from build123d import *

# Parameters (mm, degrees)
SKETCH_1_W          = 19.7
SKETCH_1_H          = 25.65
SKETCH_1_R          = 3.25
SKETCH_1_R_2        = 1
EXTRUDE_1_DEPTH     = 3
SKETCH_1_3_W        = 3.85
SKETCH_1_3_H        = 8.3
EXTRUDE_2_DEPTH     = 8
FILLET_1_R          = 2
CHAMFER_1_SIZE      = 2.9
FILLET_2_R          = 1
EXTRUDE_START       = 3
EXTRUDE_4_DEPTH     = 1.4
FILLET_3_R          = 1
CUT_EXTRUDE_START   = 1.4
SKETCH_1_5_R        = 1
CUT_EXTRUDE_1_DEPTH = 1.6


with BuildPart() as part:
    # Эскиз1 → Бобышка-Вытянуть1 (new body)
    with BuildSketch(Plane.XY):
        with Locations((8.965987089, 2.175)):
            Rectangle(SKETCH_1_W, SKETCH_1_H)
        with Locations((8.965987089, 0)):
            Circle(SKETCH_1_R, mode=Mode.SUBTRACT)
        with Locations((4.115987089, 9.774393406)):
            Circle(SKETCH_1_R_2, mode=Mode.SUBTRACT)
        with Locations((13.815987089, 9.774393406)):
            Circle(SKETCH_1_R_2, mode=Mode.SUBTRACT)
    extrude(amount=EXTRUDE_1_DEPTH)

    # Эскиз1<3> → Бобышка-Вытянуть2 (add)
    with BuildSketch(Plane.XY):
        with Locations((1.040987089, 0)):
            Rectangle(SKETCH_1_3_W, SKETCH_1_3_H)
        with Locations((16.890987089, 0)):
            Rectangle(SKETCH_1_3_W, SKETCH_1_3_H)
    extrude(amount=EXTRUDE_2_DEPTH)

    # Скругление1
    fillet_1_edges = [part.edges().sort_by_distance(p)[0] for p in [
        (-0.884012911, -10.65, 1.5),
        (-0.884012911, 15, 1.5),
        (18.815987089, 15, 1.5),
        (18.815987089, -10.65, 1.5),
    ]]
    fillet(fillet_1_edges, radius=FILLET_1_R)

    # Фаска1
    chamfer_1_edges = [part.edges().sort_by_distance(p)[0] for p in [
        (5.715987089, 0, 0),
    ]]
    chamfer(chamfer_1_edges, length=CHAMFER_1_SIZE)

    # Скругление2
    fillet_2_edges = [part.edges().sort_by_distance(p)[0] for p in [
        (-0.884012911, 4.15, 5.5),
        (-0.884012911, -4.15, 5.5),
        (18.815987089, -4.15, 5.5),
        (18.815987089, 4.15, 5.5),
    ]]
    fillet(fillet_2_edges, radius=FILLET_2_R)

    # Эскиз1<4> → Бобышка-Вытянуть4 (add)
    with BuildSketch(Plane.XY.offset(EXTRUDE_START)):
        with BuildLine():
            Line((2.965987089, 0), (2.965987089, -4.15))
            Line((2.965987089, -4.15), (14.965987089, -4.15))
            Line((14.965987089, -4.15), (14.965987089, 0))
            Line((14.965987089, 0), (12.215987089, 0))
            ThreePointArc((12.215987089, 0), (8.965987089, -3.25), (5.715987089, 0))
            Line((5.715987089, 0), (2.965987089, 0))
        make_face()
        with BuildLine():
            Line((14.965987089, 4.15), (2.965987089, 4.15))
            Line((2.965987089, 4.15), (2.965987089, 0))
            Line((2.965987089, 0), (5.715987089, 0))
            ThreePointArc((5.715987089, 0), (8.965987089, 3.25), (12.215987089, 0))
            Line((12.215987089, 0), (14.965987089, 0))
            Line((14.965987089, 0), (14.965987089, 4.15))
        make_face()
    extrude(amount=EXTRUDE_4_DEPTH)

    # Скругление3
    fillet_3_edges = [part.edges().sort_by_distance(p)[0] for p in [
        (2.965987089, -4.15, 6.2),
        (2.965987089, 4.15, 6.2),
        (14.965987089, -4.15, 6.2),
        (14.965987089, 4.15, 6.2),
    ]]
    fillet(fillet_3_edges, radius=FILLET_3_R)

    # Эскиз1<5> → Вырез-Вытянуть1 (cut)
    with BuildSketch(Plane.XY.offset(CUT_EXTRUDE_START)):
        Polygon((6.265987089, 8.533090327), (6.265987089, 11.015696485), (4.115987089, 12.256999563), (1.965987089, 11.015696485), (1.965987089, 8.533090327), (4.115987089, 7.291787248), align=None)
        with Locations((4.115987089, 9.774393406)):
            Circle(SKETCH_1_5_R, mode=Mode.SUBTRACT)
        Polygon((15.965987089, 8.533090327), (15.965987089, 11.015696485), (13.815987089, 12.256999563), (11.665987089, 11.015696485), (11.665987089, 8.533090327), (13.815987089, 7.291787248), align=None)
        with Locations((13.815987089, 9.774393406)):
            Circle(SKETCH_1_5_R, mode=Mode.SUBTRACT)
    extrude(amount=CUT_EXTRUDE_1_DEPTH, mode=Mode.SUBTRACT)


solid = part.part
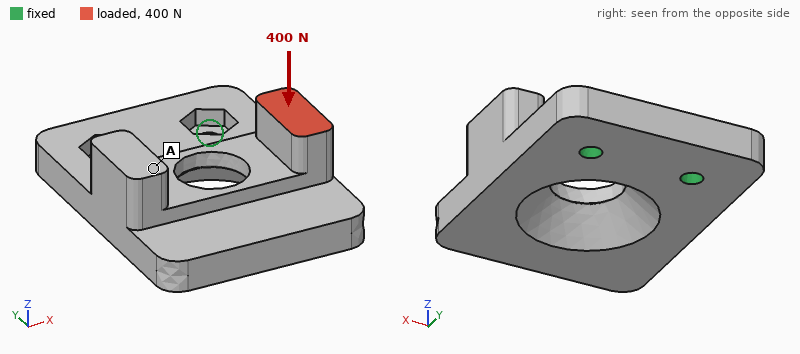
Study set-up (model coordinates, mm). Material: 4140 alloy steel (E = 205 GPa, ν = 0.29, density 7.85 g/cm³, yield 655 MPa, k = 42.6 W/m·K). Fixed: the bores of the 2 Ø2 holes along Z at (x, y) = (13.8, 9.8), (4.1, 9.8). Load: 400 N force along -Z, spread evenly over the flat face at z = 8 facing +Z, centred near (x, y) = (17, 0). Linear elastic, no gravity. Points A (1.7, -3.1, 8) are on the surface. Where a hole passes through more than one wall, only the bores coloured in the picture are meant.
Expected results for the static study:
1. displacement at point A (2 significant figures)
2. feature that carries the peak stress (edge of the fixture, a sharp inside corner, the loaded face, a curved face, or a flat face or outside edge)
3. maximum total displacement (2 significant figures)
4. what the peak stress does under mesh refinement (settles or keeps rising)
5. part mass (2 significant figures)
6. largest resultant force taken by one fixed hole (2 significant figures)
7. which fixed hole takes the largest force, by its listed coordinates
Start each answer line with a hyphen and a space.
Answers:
- 0.054 mm
- edge of the fixture
- 0.12 mm
- keeps rising
- 13 g
- 480 N
- (13.8, 9.8)
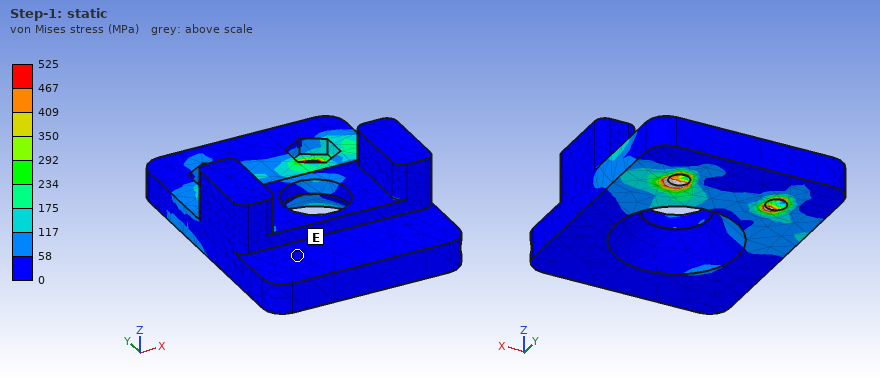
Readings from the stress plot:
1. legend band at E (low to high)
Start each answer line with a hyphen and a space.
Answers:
- 0 to 58 MPa
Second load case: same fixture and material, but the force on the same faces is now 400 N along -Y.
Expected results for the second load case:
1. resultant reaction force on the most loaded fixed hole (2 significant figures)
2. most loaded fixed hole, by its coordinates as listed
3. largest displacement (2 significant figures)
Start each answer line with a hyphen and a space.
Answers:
- 480 N
- (13.8, 9.8)
- 0.10 mm
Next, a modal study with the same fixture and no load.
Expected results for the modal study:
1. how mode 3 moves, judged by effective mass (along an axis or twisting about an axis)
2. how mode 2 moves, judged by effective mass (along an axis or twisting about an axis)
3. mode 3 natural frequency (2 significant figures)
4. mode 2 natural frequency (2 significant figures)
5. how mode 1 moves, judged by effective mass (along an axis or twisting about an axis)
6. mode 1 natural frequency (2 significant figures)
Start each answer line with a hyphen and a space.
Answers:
- along X
- twisting about Y
- 14 kHz
- 9300 Hz
- along Z
- 3600 Hz
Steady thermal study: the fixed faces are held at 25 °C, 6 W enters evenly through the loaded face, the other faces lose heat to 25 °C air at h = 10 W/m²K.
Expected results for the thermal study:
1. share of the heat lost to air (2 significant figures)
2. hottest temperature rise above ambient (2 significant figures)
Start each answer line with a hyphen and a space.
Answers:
- 5.5 %
- 65 K
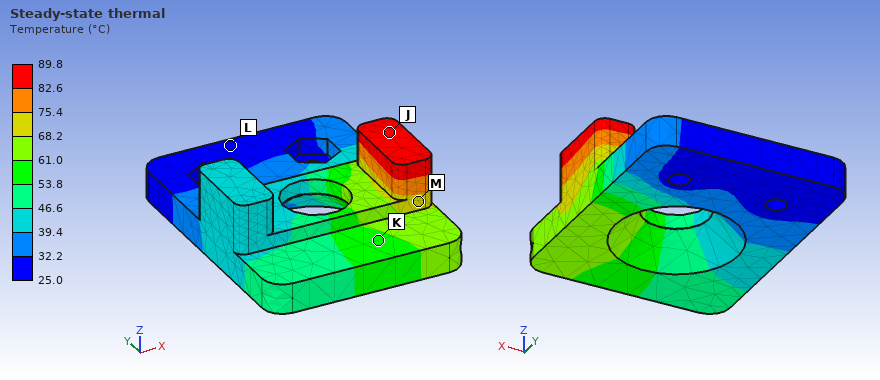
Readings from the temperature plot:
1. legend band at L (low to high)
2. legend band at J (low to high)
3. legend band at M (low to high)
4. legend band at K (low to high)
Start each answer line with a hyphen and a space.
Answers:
- 25.0 to 32.2 °C
- 82.6 to 89.8 °C
- 68.2 to 75.4 °C
- 53.8 to 61.0 °C
